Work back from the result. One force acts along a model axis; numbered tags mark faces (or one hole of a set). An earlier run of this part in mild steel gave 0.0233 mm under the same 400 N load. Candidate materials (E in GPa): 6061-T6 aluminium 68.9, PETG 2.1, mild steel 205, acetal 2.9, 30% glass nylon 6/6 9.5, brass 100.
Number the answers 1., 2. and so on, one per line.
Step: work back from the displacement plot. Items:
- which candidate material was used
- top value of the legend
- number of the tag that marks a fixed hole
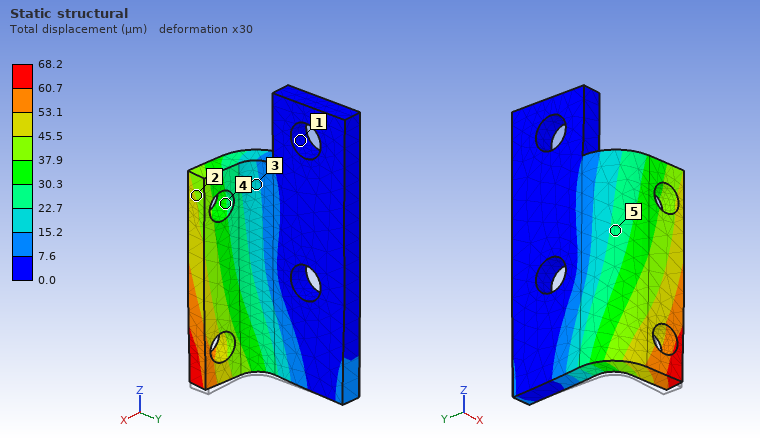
1. 6061-T6 aluminium
2. 68.2 µm
3. 1
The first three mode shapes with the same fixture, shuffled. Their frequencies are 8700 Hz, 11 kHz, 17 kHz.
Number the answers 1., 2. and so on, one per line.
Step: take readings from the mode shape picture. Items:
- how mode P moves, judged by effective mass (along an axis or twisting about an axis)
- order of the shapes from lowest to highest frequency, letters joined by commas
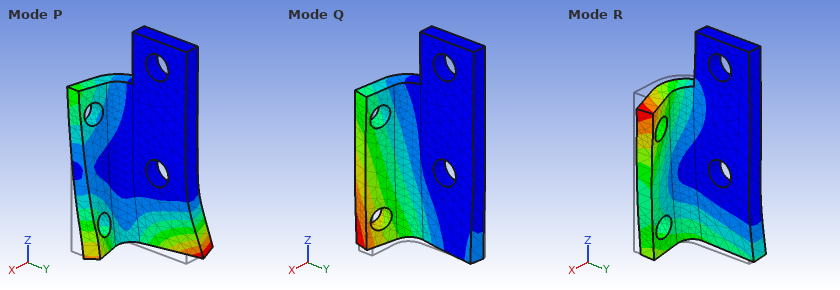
1. along X
2. Q, R, P
